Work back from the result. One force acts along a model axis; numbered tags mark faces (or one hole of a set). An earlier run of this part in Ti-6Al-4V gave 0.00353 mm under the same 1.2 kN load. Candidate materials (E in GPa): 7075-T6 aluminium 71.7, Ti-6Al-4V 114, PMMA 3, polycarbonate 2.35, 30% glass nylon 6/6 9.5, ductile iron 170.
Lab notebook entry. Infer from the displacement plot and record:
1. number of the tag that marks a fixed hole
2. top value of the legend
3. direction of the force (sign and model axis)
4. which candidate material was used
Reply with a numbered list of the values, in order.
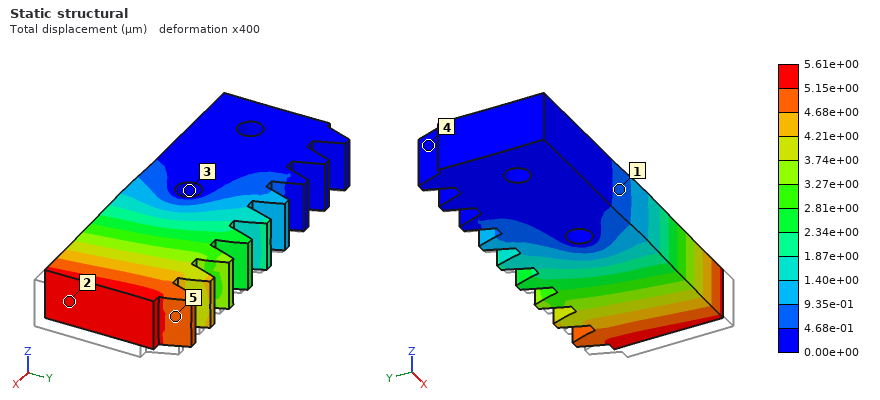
1. 3
2. 5.61e+00 µm
3. -X
4. 7075-T6 aluminium
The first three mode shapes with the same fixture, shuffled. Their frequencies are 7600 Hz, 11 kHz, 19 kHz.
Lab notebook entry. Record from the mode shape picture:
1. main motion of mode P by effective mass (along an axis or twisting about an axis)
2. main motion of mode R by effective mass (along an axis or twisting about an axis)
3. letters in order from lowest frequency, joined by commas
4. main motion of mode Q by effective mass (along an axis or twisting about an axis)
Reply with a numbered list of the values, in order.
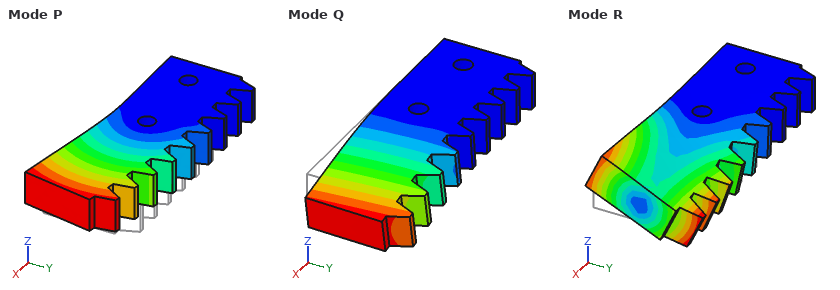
1. along Y
2. twisting about X
3. Q, P, R
4. along Z
